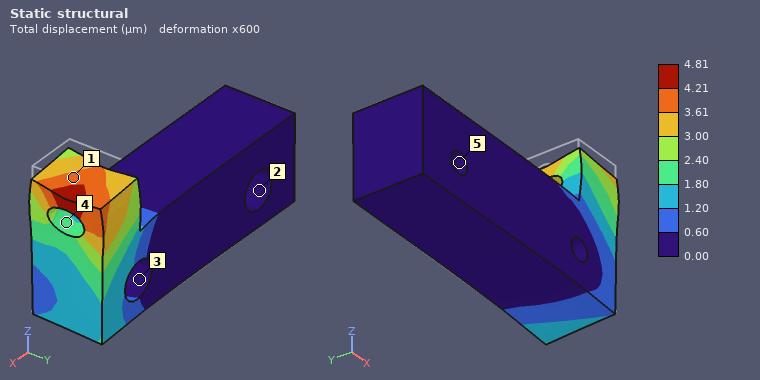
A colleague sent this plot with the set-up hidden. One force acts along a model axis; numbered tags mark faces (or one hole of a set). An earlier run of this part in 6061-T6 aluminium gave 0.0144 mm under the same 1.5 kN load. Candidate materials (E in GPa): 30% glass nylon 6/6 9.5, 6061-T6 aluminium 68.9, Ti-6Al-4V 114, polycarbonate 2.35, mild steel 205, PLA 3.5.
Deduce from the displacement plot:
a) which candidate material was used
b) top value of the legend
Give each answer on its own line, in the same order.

mild steel
4.81 µm
